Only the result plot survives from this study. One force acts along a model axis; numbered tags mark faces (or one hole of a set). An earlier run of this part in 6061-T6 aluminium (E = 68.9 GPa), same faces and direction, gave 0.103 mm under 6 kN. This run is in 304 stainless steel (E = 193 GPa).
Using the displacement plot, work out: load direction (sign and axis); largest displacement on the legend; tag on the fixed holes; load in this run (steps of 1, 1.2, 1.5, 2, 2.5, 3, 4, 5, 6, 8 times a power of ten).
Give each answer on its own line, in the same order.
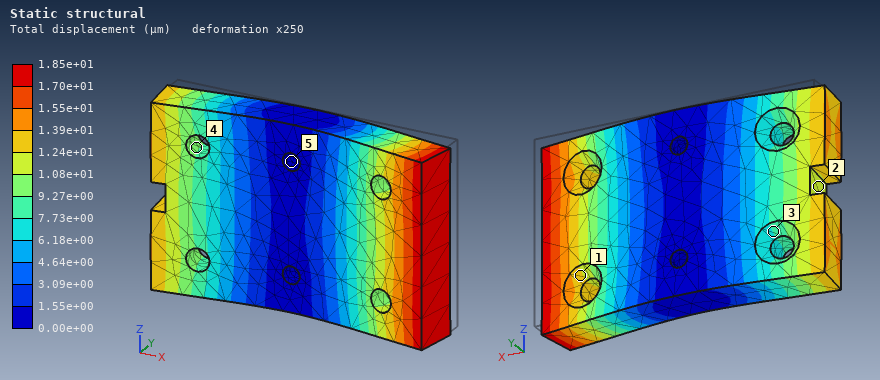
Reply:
-Y
1.85e+01 µm
5
3 kN
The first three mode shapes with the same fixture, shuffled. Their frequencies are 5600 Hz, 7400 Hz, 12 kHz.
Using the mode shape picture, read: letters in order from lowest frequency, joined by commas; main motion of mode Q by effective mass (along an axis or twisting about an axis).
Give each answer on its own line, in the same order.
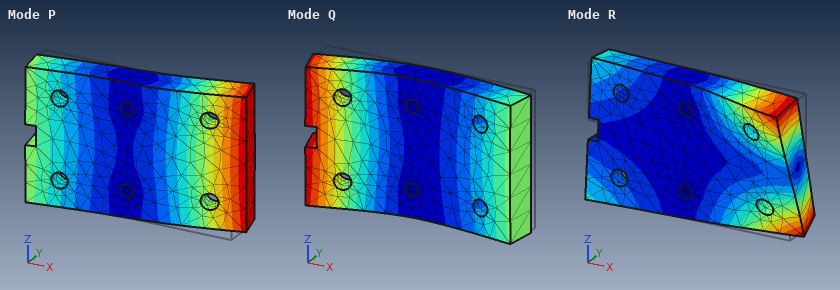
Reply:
P, Q, R
along Y
